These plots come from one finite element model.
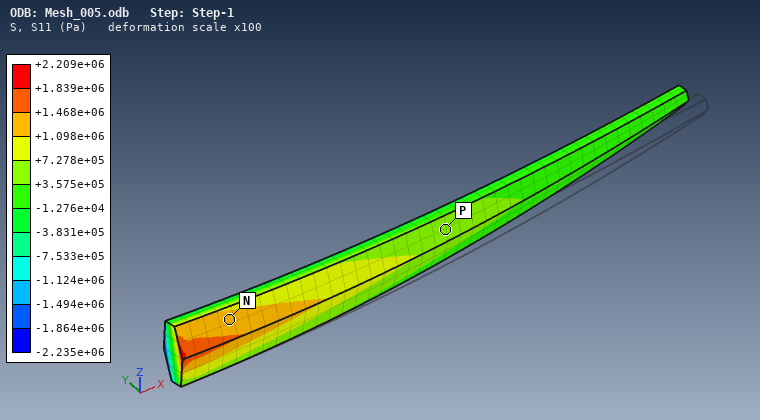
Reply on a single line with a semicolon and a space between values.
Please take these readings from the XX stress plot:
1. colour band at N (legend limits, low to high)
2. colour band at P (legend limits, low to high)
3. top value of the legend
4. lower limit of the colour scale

+1.098e+06 to +1.468e+06 Pa; +3.575e+05 to +7.278e+05 Pa; +2.209e+06 Pa; -2.235e+06 Pa
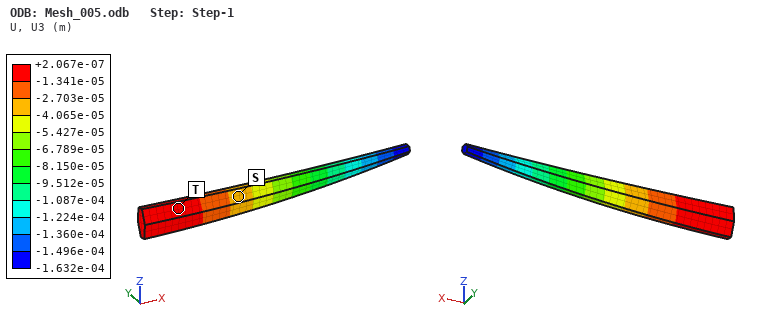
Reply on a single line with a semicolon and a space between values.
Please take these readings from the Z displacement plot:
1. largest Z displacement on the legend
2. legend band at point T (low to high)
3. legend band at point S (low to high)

+2.067e-07 m; -1.341e-05 to +2.067e-07 m; -4.065e-05 to -2.703e-05 m
